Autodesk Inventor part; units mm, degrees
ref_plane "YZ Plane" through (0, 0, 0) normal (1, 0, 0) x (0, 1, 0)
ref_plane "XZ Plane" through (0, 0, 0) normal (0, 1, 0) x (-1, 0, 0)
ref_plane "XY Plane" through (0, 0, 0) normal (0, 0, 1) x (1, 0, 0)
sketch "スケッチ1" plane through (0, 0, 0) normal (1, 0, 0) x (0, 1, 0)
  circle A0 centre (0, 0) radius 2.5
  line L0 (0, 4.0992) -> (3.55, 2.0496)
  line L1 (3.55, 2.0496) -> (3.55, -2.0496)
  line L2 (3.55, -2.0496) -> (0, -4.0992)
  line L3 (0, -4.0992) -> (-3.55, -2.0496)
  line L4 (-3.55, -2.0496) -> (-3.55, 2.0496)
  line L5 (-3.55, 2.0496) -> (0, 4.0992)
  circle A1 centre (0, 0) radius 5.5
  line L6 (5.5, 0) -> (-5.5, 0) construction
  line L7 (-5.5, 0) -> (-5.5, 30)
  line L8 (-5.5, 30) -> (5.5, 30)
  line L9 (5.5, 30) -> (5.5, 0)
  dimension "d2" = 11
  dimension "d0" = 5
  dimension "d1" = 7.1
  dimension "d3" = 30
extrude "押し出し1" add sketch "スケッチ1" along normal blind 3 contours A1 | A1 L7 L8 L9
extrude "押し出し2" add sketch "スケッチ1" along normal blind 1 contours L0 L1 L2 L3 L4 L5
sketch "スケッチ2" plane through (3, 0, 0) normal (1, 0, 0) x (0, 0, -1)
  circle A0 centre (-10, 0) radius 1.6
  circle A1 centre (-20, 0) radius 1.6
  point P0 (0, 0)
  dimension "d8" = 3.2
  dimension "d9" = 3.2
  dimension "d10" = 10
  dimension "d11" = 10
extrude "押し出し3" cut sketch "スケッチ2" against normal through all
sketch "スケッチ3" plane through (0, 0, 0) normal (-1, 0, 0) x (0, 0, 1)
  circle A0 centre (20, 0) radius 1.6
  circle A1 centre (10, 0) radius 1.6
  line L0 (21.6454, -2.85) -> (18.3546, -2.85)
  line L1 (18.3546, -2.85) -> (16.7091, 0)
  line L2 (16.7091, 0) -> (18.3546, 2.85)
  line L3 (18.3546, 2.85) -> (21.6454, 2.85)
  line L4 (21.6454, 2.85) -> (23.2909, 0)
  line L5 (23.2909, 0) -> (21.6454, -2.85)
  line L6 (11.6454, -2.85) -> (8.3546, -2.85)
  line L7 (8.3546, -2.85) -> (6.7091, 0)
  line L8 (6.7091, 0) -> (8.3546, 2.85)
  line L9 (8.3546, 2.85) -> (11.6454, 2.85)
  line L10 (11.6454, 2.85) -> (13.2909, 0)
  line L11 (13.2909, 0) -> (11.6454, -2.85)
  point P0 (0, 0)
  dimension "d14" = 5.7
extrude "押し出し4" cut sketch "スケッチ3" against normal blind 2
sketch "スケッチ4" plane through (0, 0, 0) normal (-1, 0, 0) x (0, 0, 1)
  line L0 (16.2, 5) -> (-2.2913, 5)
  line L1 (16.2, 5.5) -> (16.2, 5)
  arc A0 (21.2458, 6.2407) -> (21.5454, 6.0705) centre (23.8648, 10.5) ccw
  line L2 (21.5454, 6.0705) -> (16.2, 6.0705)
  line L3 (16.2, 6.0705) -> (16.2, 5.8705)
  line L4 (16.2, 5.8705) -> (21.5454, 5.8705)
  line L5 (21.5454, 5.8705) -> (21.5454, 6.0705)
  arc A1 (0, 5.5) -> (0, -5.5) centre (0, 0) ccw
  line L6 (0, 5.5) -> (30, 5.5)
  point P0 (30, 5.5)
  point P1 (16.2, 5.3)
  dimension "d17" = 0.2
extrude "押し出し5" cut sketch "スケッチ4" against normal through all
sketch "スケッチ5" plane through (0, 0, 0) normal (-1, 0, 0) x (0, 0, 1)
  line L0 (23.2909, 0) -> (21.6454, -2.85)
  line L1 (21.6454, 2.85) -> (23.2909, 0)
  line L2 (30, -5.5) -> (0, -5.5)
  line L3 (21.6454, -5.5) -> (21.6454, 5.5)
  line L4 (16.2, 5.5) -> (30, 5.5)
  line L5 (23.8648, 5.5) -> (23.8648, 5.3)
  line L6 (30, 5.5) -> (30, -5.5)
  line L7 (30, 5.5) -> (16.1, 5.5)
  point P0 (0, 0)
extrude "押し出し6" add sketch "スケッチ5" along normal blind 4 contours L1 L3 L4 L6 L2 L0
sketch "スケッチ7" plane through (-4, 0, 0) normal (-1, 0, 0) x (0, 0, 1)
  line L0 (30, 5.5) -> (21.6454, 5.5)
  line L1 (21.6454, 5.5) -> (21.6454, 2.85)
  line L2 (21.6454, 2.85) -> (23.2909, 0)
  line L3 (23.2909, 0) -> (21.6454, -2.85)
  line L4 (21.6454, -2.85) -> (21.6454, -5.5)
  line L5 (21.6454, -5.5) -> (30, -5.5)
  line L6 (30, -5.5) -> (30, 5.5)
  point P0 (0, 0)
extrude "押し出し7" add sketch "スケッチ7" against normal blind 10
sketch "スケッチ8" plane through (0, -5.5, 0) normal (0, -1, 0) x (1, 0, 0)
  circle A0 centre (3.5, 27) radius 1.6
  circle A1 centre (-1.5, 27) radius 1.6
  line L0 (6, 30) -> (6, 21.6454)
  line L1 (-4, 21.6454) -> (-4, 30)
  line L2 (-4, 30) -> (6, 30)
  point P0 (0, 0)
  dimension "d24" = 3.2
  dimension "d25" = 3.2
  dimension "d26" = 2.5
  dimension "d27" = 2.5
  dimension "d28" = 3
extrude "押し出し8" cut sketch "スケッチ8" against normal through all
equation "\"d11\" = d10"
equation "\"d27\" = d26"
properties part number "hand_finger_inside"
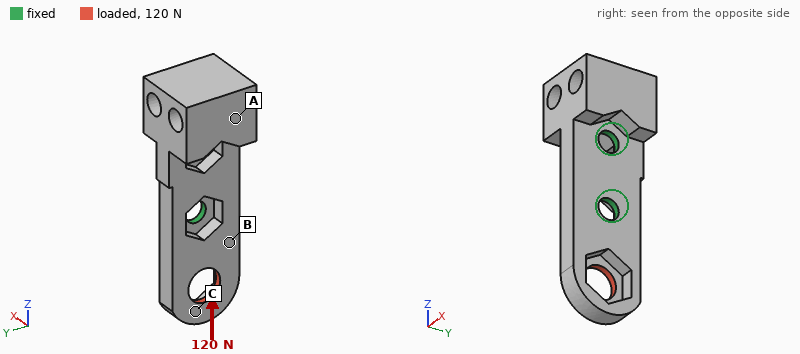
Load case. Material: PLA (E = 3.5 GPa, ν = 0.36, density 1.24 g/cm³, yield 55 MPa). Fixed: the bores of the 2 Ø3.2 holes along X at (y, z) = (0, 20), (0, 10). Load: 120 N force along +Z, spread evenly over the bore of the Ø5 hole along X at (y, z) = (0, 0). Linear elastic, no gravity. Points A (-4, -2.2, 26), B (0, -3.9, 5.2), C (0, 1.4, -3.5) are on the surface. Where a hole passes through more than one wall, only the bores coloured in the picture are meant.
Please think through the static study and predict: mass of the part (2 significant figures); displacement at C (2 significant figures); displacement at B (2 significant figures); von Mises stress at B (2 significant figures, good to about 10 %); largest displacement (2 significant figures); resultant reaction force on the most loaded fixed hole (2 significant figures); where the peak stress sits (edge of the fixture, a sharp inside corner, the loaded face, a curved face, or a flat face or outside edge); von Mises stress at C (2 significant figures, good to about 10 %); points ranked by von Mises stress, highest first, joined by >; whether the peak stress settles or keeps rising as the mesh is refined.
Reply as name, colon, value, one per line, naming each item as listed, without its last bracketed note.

mass of the part: 1.6 g
displacement at C: 0.29 mm
displacement at B: 0.077 mm
von Mises stress at B: 15 MPa
largest displacement: 0.35 mm
resultant reaction force on the most loaded fixed hole: 64 N
where the peak stress sits: edge of the fixture
von Mises stress at C: 8.1 MPa
points ranked by von Mises stress, highest first, joined by >: B > C > A
whether the peak stress settles or keeps rising as the mesh is refined: keeps rising
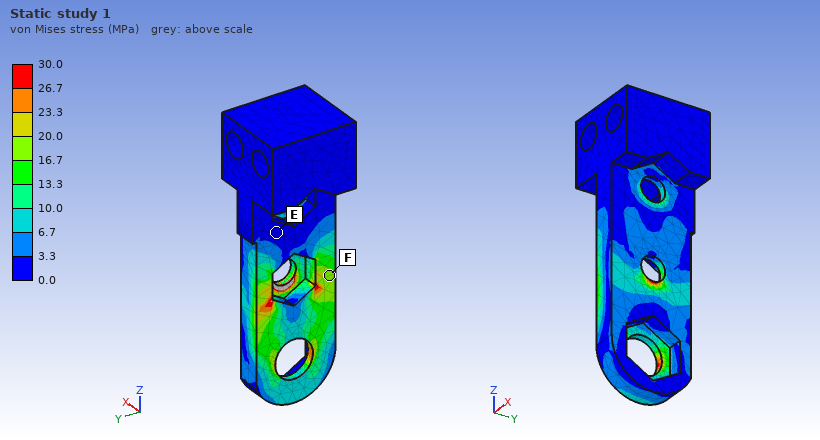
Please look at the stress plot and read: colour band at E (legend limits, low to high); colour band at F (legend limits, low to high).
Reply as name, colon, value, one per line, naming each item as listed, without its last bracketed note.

colour band at E: 0.0 to 3.3 MPa
colour band at F: 16.7 to 20.0 MPa
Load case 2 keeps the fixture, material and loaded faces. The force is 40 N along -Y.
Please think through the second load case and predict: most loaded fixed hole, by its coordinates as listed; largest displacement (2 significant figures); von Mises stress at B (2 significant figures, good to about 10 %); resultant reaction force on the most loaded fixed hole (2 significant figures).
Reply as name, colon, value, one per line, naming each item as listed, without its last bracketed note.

most loaded fixed hole, by its coordinates as listed: (0, 10)
largest displacement: 0.13 mm
von Mises stress at B: 4.5 MPa
resultant reaction force on the most loaded fixed hole: 63 N
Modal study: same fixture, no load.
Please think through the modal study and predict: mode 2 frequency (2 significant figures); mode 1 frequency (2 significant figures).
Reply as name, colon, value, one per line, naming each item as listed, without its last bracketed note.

mode 2 frequency: 3300 Hz
mode 1 frequency: 3200 Hz
